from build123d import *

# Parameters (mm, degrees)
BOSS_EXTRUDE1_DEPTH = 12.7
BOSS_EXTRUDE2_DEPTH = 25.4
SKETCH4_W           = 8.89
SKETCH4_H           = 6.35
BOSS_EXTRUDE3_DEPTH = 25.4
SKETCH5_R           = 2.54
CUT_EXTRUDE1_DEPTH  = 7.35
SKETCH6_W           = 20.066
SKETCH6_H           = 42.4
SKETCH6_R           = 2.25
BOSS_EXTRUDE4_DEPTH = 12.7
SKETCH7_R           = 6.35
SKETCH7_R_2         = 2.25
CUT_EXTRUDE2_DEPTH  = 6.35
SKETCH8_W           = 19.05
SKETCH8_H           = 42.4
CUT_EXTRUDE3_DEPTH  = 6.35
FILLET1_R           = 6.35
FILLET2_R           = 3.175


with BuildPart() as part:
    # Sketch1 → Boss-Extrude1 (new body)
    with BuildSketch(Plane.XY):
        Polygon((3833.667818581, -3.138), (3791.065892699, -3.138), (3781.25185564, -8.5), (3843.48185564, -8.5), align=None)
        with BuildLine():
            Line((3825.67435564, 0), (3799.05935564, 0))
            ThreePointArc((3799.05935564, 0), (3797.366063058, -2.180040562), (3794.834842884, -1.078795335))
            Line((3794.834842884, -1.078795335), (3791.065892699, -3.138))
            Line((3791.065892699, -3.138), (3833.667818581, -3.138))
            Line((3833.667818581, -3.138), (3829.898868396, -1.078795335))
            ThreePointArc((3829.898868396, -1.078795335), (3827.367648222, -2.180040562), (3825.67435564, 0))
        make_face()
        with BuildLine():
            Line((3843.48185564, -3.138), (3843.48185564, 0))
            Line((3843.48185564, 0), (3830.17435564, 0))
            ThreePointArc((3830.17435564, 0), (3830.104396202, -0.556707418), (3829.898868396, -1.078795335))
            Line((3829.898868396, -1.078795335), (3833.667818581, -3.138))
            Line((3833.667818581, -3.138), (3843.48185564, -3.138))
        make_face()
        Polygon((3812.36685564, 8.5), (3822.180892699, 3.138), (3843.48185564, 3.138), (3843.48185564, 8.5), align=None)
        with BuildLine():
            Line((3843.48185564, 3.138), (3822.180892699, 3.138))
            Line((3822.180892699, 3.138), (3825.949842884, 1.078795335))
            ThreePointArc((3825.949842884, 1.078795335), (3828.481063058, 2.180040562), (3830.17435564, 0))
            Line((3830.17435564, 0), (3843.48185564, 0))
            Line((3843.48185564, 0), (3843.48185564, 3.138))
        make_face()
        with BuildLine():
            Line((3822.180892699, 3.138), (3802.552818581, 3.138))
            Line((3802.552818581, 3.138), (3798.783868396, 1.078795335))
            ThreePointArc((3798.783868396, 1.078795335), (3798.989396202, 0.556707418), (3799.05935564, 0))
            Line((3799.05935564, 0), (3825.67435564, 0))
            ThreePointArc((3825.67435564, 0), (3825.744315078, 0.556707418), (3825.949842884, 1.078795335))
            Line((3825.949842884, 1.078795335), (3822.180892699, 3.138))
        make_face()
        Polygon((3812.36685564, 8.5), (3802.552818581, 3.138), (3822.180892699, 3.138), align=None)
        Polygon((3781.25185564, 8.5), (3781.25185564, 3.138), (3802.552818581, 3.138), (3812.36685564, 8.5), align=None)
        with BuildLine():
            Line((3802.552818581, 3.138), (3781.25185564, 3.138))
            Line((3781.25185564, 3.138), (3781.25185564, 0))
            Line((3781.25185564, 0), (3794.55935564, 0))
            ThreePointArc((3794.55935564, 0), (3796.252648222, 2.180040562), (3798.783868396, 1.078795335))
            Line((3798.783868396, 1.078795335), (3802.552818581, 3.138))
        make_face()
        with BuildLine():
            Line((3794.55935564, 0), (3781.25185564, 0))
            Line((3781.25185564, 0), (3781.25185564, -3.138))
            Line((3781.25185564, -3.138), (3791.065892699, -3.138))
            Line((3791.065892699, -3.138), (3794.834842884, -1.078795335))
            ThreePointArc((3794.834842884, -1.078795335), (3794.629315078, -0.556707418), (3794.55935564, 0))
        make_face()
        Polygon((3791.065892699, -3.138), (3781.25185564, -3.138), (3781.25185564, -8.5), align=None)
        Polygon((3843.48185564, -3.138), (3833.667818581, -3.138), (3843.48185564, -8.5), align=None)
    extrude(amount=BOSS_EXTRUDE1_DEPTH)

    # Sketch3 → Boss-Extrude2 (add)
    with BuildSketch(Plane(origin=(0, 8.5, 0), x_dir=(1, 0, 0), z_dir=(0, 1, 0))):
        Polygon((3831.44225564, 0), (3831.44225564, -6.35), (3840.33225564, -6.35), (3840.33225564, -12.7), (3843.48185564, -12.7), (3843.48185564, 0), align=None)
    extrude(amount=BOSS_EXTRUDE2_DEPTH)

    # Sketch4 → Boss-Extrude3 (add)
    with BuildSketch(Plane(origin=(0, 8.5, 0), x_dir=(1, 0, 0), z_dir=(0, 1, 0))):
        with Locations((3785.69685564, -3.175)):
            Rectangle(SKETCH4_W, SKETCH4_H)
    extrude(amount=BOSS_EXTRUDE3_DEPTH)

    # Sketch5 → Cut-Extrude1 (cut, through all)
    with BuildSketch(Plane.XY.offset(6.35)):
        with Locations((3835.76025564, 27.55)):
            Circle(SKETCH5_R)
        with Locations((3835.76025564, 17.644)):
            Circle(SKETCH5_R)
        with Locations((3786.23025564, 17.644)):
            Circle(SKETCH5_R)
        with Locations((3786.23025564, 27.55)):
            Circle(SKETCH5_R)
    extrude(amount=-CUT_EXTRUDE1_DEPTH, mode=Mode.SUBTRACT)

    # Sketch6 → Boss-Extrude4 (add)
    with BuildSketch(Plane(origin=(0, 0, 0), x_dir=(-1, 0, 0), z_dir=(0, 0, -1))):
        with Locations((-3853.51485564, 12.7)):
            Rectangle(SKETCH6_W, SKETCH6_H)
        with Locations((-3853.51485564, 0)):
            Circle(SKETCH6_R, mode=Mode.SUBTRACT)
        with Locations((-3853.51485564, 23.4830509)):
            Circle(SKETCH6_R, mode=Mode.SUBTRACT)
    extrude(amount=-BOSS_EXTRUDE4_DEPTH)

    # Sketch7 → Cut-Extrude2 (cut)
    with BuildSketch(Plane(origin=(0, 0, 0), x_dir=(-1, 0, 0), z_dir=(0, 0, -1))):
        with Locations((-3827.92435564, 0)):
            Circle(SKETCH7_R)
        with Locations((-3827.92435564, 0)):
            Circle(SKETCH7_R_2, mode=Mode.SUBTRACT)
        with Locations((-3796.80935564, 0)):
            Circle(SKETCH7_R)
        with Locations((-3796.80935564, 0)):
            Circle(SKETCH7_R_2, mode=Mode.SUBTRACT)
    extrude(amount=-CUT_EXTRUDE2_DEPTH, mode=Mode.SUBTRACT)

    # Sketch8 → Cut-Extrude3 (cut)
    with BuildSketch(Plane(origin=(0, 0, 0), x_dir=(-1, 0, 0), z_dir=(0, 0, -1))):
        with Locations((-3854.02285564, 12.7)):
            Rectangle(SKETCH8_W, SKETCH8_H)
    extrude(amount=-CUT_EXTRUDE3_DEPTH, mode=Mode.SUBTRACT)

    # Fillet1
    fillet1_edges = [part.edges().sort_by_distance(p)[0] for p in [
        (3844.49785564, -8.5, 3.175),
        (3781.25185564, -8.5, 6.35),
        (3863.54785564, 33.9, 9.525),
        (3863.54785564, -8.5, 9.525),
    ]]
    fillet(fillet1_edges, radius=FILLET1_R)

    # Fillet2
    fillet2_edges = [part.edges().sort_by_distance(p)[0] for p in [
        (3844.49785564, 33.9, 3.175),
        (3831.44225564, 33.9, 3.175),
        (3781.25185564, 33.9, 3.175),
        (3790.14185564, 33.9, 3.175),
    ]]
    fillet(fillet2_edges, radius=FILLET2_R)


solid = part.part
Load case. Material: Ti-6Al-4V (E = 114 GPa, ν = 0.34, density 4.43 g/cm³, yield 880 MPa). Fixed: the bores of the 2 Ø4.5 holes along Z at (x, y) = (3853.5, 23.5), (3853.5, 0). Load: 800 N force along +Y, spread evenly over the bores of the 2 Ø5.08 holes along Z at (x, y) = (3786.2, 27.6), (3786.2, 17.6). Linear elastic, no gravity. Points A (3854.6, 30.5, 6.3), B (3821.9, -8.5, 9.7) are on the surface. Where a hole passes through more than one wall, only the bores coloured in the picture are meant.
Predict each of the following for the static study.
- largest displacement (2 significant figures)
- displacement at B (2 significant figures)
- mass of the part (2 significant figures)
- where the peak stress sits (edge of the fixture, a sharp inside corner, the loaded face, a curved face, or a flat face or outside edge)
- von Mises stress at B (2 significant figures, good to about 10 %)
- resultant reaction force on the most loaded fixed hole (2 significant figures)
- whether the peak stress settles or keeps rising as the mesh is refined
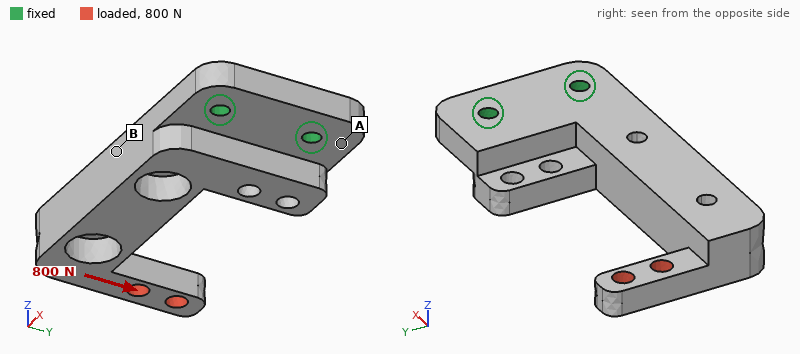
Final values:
0.20 mm
0.042 mm
89 g
a sharp inside corner
46 MPa
2.3 kN
keeps rising
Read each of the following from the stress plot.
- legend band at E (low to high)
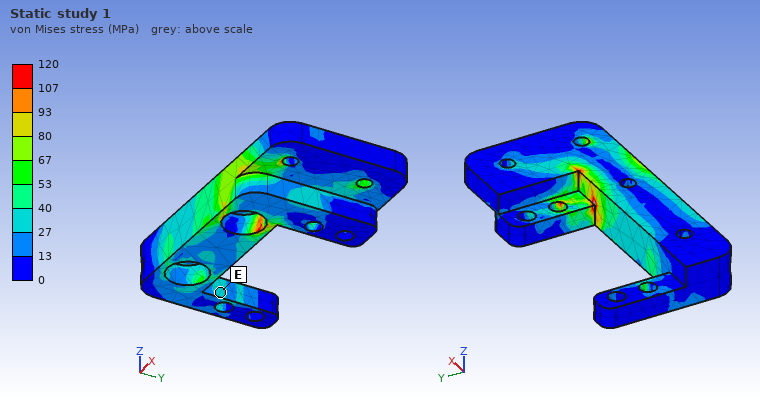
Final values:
27 to 40 MPa
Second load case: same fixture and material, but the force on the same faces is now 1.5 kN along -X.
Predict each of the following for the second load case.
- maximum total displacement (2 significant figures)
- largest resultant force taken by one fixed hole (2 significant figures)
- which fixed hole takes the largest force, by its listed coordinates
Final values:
0.37 mm
1.5 kN
(3853.5, 23.5)
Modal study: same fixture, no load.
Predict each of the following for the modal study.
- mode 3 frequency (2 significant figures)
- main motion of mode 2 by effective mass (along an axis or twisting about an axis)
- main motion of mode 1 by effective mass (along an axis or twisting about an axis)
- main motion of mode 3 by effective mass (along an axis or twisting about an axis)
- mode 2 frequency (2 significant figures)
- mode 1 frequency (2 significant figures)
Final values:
4000 Hz
along Y
along Z
twisting about X
2500 Hz
1100 Hz
